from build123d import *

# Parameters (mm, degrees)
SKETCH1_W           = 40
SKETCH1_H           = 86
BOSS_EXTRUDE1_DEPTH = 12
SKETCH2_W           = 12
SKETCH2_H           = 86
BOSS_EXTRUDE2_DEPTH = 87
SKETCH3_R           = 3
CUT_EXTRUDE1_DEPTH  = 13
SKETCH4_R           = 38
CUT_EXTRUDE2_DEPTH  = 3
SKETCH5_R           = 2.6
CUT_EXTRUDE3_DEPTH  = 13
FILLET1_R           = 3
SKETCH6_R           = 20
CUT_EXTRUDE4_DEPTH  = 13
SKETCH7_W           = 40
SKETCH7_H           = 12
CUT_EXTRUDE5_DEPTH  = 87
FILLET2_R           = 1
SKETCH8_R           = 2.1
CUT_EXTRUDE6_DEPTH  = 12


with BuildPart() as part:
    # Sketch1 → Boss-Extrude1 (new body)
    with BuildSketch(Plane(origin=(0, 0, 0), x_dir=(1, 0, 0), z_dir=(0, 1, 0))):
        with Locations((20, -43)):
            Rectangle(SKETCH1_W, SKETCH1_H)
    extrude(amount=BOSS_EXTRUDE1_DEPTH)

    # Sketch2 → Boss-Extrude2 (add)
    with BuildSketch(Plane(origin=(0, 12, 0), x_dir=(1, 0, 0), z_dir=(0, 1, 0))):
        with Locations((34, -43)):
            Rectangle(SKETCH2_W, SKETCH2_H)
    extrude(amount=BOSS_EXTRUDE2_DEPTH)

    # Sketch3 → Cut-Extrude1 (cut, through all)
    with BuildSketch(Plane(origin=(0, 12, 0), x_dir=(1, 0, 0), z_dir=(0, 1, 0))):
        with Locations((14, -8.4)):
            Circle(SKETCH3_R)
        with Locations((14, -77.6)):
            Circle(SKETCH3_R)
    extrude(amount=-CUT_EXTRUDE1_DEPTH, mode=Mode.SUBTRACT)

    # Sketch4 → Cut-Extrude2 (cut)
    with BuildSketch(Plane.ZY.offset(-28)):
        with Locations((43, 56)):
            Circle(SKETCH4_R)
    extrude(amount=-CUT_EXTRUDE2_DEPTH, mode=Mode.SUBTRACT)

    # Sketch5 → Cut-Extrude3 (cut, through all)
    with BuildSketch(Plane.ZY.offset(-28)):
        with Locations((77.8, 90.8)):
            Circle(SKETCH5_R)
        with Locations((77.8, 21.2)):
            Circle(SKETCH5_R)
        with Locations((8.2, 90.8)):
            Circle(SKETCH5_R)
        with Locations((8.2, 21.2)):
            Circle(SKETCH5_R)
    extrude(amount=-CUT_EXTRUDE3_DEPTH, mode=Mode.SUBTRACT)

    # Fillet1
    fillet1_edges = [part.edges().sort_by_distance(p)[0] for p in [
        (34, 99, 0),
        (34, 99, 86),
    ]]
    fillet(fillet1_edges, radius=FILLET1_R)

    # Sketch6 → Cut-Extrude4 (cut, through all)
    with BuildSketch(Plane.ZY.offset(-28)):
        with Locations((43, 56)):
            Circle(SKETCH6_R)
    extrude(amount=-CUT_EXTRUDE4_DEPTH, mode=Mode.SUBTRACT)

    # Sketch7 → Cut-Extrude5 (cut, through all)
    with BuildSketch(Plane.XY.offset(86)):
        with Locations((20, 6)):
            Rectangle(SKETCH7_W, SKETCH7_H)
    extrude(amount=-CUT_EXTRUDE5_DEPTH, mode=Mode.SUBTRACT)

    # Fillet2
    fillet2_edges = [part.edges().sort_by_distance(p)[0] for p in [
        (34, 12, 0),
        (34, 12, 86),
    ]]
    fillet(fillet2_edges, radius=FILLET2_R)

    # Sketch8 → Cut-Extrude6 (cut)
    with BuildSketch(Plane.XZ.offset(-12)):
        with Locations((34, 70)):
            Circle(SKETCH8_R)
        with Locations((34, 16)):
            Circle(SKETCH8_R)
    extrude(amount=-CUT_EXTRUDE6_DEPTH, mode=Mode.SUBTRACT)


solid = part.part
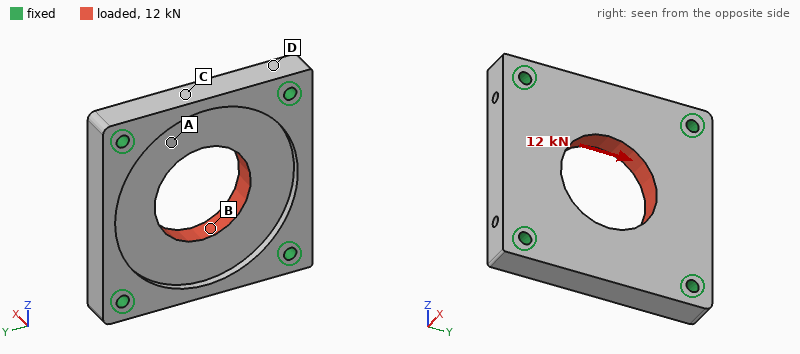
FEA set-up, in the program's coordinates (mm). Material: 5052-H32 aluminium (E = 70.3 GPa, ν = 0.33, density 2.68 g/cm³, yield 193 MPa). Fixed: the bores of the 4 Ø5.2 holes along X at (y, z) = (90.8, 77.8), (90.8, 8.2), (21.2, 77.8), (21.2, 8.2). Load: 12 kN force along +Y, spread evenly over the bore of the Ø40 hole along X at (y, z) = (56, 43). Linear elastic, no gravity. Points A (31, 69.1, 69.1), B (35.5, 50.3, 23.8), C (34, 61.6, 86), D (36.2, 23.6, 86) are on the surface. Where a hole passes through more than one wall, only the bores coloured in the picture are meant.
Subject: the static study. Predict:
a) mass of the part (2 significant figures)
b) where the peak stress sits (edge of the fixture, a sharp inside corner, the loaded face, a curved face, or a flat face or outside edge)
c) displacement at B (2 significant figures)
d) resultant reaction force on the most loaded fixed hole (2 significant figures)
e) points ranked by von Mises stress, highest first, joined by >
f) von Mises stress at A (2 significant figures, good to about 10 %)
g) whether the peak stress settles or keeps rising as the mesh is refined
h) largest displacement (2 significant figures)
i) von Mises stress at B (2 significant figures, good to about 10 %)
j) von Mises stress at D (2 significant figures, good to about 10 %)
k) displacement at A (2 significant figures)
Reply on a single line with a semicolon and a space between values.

170 g; edge of the fixture; 7.5 µm; 3.2 kN; B > A > D > C; 15 MPa; keeps rising; 13 µm; 21 MPa; 7.9 MPa; 5.4 µm
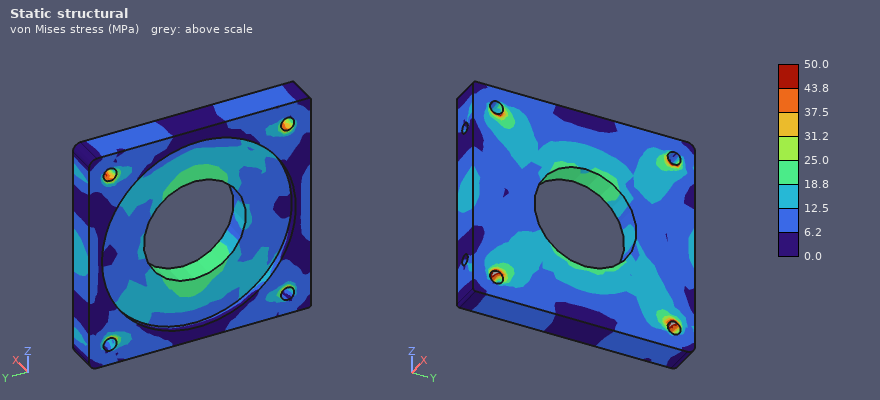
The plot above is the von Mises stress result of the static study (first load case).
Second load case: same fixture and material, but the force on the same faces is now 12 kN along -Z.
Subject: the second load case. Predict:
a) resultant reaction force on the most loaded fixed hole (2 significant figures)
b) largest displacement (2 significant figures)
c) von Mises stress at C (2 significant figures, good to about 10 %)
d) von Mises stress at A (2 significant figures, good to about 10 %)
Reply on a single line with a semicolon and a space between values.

3.2 kN; 13 µm; 13 MPa; 13 MPa
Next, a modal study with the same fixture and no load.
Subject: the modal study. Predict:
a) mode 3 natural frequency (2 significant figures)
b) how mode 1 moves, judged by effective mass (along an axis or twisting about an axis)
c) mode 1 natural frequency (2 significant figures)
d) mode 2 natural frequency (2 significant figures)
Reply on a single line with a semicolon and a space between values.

11 kHz; along X; 8600 Hz; 11 kHz
